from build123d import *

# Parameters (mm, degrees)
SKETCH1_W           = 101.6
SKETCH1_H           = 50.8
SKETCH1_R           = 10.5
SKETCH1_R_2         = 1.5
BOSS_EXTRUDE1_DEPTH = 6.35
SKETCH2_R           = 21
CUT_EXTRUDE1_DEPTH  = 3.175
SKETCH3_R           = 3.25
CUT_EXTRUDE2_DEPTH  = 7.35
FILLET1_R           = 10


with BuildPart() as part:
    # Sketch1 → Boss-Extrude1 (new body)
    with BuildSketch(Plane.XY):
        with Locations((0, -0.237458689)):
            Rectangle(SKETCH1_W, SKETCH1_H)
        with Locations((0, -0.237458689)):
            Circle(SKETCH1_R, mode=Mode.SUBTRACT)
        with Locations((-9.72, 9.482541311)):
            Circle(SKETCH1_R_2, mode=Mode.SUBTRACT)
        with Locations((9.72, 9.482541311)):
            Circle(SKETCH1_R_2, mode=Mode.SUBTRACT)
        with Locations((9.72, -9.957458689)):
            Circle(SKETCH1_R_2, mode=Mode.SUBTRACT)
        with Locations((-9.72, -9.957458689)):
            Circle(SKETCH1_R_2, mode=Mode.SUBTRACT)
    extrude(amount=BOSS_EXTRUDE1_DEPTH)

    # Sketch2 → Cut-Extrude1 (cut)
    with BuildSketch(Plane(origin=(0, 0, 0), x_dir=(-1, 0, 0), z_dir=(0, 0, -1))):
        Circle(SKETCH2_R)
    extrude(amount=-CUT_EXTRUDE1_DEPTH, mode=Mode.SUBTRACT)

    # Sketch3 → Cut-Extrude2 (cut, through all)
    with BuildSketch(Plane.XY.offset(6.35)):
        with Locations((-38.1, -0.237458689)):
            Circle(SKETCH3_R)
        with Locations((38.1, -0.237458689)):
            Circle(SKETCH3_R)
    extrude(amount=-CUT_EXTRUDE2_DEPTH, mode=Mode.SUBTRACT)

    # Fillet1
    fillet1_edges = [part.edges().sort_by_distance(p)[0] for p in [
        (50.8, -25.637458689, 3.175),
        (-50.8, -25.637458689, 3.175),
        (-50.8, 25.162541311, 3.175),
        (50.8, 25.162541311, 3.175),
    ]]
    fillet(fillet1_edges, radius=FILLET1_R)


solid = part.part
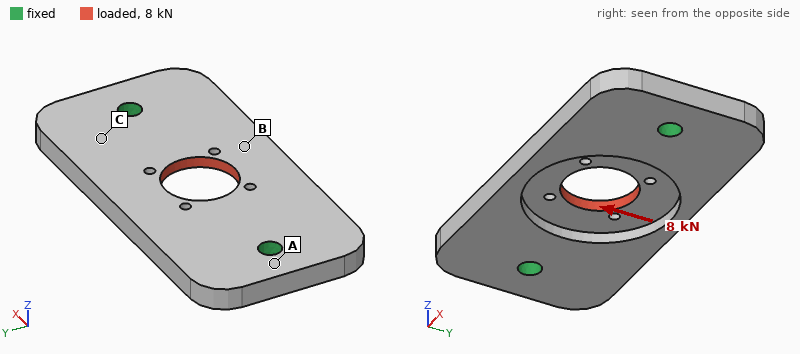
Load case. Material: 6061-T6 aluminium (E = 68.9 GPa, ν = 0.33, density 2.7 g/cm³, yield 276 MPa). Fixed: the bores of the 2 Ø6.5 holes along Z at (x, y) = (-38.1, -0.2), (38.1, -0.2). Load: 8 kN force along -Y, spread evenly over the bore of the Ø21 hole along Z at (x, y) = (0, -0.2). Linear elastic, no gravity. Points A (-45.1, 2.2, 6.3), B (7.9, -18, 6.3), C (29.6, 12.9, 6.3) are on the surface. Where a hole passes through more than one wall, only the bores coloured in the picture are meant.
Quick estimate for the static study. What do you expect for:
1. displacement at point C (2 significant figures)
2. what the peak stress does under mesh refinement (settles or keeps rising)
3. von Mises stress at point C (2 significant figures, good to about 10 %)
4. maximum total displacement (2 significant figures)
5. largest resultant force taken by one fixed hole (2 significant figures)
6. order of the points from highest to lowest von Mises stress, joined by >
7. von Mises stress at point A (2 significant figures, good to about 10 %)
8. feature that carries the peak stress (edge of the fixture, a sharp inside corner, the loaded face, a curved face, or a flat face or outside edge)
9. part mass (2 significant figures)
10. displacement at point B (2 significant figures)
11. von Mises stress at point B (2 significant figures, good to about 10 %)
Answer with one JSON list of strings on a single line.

["18 µm", "keeps rising", "32 MPa", "60 µm", "4.0 kN", "B > C > A", "12 MPa", "edge of the fixture", "71 g", "46 µm", "49 MPa"]
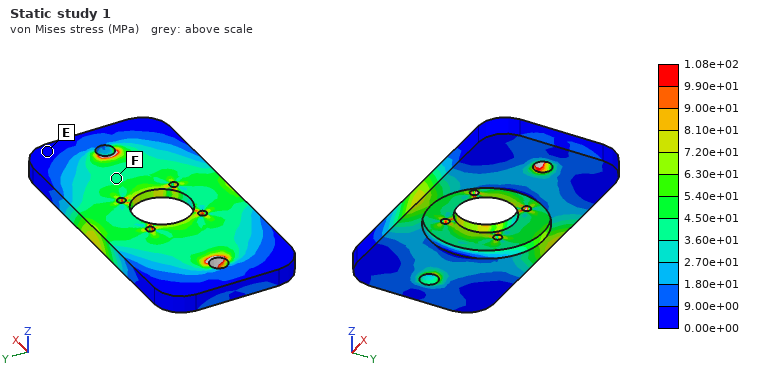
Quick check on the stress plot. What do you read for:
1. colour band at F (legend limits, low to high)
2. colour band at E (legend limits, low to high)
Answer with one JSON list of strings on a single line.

["3.60e+01 to 4.50e+01 MPa", "0.00e+00 to 9.00e+00 MPa"]
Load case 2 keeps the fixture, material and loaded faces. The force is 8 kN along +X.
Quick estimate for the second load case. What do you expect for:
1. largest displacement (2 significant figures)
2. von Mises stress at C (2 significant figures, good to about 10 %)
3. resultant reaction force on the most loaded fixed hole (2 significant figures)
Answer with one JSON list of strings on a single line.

["21 µm", "17 MPa", "4.0 kN"]
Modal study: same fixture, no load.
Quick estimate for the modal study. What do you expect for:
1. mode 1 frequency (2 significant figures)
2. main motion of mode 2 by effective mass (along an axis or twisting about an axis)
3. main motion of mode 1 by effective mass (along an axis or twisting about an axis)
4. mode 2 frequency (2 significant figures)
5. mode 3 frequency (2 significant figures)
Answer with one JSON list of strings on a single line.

["4500 Hz", "along Z", "twisting about X", "4900 Hz", "7700 Hz"]
